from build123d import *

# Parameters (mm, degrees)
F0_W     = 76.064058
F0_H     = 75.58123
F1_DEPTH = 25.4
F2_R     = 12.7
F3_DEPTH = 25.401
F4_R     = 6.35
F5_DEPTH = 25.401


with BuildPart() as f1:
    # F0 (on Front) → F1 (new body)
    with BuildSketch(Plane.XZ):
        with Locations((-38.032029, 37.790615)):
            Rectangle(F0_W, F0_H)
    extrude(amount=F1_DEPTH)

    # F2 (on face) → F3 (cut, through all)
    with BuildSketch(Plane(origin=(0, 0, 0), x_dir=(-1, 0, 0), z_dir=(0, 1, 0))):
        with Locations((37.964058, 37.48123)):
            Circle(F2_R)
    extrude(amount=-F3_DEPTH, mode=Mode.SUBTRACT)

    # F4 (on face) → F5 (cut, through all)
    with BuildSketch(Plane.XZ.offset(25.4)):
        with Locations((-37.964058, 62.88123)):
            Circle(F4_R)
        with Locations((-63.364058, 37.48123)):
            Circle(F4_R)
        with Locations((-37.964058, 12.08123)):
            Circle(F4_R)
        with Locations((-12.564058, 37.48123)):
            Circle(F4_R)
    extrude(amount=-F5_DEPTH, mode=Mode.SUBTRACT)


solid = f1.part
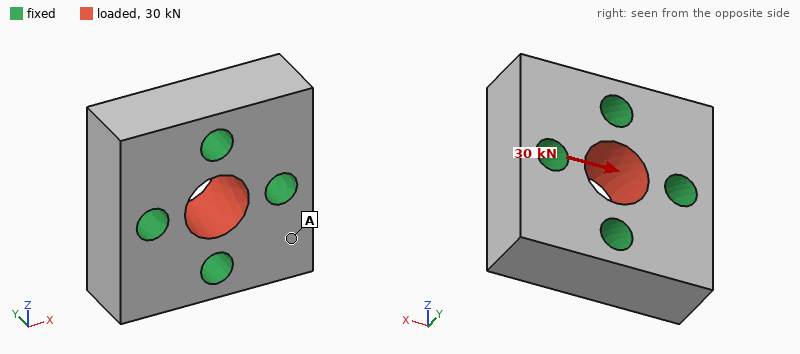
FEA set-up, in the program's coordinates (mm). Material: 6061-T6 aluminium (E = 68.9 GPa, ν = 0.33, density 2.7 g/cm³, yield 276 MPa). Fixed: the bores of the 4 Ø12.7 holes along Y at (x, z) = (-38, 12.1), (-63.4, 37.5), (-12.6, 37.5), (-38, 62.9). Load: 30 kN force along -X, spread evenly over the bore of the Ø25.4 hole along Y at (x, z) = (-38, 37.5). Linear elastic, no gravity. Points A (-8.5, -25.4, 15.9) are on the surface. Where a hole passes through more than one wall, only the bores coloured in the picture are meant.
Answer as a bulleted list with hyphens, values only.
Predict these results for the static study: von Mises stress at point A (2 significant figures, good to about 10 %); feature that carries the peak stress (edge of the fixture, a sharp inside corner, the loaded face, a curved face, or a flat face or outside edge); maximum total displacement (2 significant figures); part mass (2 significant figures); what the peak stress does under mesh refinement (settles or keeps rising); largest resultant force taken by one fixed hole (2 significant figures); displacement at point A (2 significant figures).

- 2.7 MPa
- edge of the fixture
- 3.6 µm
- 320 g
- keeps rising
- 8.9 kN
- 0.96 µm
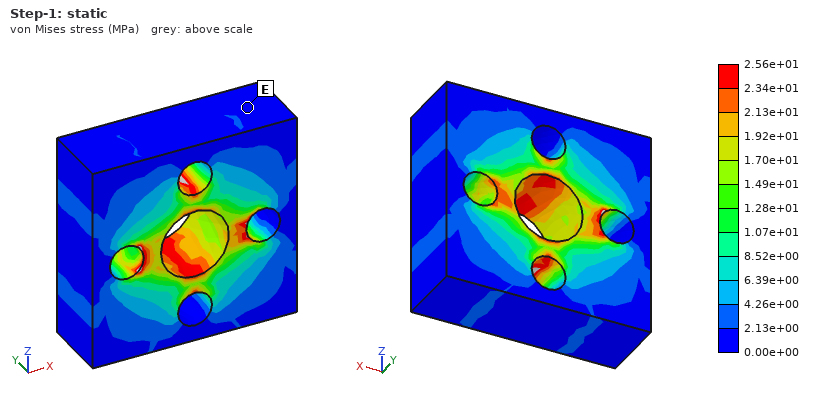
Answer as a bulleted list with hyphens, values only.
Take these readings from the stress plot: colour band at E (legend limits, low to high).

- 0.00e+00 to 2.13e+00 MPa
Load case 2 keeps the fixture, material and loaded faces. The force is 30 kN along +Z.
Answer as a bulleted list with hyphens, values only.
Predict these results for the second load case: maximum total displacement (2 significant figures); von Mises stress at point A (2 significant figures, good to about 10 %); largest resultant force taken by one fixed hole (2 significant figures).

- 3.6 µm
- 2.5 MPa
- 8.9 kN
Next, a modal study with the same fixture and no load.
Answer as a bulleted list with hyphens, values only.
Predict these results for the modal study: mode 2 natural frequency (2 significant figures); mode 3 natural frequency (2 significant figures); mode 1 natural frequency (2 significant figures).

- 21 kHz
- 21 kHz
- 20 kHz
